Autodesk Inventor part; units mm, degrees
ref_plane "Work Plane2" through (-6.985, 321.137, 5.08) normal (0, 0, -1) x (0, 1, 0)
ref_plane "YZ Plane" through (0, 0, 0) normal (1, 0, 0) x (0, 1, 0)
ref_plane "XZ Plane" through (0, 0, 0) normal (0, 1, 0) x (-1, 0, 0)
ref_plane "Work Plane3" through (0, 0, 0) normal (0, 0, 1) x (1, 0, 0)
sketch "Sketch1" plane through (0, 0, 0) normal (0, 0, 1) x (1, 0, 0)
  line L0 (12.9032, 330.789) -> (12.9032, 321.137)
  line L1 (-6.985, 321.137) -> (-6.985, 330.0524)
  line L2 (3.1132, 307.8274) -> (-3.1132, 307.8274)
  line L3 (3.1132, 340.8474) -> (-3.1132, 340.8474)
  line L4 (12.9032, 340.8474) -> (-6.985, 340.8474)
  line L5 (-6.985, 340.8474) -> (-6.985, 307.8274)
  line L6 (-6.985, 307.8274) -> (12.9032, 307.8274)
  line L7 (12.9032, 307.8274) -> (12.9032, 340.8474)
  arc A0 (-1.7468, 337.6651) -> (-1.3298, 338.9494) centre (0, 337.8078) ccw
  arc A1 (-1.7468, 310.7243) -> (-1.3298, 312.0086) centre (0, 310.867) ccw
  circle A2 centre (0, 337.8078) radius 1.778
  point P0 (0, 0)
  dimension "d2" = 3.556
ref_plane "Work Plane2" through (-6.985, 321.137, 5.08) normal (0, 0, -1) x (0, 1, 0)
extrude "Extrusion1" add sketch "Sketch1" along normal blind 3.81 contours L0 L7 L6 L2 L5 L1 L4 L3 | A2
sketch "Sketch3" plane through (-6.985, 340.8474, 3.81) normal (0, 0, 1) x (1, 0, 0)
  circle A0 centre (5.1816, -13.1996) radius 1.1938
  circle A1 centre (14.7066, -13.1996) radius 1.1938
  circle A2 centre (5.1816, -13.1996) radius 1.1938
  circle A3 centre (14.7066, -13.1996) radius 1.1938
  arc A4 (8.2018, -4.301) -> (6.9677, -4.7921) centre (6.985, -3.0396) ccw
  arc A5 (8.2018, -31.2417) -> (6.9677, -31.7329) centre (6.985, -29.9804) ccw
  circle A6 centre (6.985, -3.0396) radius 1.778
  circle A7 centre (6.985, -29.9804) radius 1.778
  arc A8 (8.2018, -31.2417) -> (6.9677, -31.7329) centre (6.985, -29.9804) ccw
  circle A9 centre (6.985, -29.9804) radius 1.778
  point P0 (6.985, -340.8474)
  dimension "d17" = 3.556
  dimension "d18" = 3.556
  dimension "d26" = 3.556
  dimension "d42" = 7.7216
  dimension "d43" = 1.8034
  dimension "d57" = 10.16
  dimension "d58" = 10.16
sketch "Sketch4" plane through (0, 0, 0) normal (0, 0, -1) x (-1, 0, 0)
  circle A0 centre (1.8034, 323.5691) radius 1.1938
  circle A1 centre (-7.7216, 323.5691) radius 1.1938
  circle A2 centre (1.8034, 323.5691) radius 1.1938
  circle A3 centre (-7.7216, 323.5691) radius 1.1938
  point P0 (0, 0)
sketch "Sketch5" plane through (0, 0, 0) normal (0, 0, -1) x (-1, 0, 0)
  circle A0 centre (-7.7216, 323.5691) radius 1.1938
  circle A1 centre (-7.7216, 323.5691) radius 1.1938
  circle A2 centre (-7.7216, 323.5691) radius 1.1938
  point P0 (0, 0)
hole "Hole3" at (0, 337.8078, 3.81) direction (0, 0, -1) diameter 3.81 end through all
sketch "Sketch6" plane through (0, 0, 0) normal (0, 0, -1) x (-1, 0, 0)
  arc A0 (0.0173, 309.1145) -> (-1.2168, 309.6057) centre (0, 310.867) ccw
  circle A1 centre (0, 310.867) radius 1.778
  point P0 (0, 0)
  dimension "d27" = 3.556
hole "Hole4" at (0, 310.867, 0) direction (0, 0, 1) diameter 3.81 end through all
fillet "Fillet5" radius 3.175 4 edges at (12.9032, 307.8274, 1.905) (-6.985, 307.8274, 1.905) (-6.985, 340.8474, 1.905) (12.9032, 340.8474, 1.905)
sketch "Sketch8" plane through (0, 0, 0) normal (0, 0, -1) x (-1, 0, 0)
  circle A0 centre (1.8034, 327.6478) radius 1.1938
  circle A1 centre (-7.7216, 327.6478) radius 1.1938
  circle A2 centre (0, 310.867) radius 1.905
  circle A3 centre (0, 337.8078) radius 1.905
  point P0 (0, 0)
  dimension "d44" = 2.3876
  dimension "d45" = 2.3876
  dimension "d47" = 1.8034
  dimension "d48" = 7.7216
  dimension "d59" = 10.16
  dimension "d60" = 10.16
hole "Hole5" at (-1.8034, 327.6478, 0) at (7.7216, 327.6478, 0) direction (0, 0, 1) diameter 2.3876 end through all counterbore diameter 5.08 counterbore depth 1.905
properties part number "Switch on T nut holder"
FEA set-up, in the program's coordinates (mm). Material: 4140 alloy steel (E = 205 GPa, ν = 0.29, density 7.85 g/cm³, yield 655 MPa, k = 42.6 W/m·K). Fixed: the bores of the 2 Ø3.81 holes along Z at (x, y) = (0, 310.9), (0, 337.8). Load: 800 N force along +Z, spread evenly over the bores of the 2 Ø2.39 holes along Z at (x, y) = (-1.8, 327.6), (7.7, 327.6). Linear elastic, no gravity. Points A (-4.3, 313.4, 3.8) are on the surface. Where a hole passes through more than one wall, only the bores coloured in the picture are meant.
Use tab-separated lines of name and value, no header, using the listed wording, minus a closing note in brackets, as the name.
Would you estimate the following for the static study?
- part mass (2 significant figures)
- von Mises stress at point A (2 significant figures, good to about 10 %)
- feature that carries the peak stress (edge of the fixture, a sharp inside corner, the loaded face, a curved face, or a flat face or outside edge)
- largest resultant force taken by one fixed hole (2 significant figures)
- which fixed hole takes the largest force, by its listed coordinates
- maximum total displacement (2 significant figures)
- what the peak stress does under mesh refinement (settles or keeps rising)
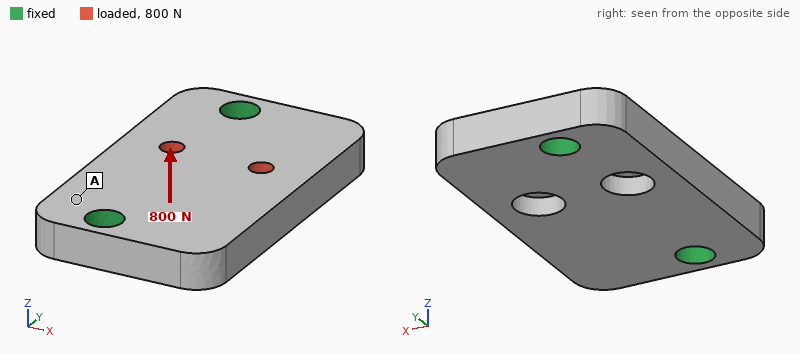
part mass	18 g
von Mises stress at point A	20 MPa
feature that carries the peak stress	edge of the fixture
largest resultant force taken by one fixed hole	550 N
which fixed hole takes the largest force, by its listed coordinates	(0, 337.8)
maximum total displacement	12 µm
what the peak stress does under mesh refinement	keeps rising
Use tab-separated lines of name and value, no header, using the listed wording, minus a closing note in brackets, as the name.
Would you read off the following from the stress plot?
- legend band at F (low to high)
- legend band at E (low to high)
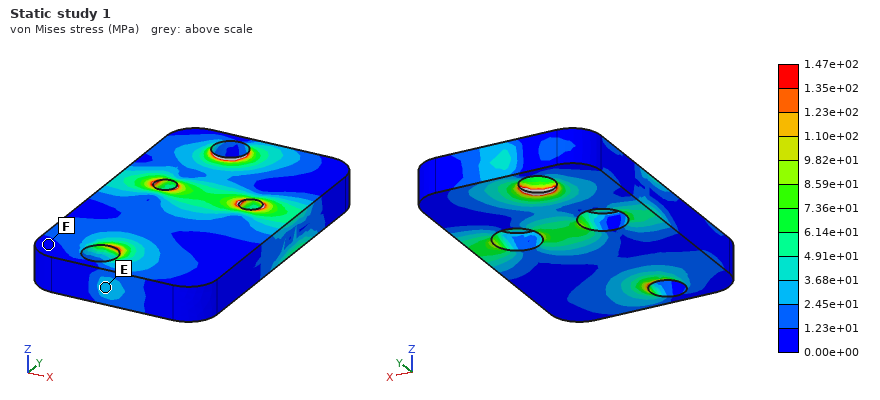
legend band at F	0.00e+00 to 1.23e+01 MPa
legend band at E	2.45e+01 to 3.68e+01 MPa
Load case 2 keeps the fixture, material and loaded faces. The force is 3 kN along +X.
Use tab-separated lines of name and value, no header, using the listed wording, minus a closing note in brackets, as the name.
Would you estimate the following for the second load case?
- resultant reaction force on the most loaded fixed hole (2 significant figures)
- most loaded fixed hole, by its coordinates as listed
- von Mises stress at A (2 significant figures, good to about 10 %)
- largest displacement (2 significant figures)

resultant reaction force on the most loaded fixed hole	1.9 kN
most loaded fixed hole, by its coordinates as listed	(0, 337.8)
von Mises stress at A	28 MPa
largest displacement	11 µm
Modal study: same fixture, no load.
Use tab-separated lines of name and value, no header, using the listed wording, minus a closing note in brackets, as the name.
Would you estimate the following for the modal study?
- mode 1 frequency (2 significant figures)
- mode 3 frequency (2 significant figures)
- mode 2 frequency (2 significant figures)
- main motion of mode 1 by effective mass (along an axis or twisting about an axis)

mode 1 frequency	15 kHz
mode 3 frequency	26 kHz
mode 2 frequency	26 kHz
main motion of mode 1 by effective mass	along Z
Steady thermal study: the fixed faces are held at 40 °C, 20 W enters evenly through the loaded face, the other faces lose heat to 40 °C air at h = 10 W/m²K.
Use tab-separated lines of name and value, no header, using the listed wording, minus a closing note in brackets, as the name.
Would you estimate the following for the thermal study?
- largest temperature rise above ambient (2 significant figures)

largest temperature rise above ambient	64 K
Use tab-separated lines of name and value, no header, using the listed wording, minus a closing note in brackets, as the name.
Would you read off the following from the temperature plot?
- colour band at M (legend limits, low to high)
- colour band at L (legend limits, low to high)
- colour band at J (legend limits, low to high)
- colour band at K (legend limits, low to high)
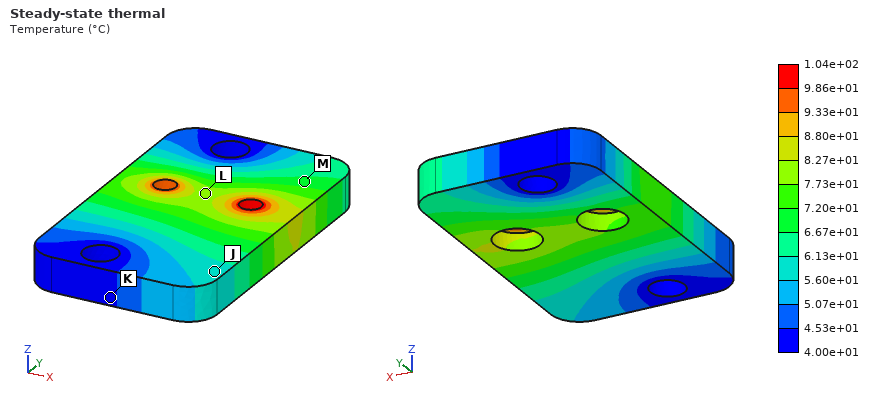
colour band at M	6.67e+01 to 7.20e+01 °C
colour band at L	7.73e+01 to 8.27e+01 °C
colour band at J	5.60e+01 to 6.13e+01 °C
colour band at K	4.00e+01 to 4.53e+01 °C
